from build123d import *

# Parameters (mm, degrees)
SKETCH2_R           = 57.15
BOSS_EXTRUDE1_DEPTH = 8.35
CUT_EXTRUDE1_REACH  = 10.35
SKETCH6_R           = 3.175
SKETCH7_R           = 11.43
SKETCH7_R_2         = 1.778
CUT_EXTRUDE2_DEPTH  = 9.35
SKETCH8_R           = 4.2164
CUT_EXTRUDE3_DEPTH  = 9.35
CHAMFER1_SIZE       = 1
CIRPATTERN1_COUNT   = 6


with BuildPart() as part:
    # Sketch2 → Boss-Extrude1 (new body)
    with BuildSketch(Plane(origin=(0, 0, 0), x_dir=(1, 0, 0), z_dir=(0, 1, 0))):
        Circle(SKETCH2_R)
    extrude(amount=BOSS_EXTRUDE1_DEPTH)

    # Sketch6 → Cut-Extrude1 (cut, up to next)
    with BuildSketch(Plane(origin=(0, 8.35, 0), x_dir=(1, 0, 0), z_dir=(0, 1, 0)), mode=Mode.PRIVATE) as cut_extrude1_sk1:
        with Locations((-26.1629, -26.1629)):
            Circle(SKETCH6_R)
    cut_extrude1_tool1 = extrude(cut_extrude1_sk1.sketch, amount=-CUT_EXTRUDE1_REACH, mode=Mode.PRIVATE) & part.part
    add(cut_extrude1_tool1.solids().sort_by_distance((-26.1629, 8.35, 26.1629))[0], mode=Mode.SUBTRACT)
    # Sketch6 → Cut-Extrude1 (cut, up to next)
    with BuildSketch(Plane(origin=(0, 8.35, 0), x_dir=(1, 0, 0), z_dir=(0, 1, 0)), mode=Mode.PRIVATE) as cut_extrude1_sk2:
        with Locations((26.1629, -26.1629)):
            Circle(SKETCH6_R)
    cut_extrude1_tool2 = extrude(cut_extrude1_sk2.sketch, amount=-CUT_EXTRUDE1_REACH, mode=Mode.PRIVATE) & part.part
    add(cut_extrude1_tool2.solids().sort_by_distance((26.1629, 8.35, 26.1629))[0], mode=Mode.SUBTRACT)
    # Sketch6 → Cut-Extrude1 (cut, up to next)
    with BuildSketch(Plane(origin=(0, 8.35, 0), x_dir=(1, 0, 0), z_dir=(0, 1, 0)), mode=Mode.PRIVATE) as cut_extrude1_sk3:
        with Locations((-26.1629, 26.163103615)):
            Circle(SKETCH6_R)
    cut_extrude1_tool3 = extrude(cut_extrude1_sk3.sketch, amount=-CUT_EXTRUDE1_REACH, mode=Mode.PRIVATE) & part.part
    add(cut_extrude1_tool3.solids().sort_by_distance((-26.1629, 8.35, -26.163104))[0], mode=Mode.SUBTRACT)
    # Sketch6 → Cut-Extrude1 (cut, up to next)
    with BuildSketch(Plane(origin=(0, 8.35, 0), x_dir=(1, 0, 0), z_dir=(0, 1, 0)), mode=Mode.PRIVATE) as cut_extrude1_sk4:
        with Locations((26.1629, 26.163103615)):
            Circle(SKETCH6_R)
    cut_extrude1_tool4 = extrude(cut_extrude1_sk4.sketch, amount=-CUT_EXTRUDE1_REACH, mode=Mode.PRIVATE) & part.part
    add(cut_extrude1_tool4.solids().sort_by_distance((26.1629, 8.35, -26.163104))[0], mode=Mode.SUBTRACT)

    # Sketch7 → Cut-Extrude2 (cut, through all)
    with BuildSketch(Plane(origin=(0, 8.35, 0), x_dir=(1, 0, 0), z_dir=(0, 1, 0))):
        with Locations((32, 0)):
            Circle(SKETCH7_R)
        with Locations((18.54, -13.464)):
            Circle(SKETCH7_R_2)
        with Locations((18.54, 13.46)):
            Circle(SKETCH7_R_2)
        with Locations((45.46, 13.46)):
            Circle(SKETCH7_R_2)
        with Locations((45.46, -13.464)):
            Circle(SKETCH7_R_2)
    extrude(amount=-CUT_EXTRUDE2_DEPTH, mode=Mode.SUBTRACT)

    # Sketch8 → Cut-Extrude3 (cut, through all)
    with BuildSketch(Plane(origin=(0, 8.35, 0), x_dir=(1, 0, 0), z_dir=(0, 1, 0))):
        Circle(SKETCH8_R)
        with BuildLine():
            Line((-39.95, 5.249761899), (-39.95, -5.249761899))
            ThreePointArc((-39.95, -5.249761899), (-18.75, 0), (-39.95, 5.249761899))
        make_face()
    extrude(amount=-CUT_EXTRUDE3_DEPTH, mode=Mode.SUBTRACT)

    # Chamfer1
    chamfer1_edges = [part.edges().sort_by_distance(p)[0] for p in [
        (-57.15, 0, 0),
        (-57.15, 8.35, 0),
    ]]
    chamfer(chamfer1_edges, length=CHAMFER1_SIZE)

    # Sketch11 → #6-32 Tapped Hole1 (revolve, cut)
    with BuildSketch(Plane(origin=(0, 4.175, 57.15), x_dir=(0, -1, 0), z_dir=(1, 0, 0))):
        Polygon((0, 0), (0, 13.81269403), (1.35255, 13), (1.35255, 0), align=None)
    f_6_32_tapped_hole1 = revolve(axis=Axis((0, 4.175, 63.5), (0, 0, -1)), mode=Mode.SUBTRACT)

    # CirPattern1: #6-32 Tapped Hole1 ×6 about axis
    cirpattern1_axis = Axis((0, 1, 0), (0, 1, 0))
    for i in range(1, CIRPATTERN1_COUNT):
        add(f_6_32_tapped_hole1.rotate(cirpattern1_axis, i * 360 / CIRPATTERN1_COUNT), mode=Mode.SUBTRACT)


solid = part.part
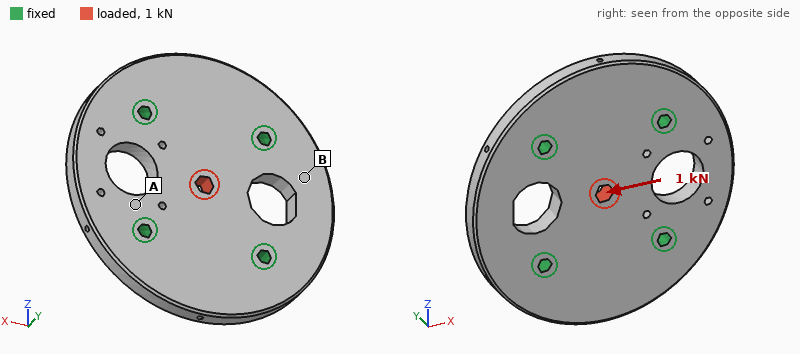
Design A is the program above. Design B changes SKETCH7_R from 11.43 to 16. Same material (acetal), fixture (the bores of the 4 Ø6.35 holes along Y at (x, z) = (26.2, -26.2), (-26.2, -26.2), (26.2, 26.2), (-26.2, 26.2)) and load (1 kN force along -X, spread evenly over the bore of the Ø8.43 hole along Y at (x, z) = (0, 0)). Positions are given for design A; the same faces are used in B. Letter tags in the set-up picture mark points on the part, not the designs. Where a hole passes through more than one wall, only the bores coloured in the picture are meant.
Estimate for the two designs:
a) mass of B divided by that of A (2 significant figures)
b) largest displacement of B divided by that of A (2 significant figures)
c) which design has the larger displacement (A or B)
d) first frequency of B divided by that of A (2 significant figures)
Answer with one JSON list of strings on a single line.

["0.96", "1.2", "B", "0.99"]
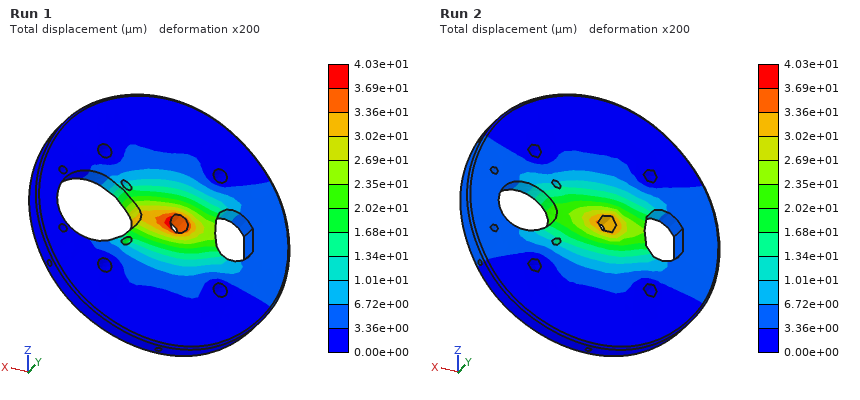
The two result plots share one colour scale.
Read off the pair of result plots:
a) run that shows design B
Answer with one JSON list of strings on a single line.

["Run 1"]
